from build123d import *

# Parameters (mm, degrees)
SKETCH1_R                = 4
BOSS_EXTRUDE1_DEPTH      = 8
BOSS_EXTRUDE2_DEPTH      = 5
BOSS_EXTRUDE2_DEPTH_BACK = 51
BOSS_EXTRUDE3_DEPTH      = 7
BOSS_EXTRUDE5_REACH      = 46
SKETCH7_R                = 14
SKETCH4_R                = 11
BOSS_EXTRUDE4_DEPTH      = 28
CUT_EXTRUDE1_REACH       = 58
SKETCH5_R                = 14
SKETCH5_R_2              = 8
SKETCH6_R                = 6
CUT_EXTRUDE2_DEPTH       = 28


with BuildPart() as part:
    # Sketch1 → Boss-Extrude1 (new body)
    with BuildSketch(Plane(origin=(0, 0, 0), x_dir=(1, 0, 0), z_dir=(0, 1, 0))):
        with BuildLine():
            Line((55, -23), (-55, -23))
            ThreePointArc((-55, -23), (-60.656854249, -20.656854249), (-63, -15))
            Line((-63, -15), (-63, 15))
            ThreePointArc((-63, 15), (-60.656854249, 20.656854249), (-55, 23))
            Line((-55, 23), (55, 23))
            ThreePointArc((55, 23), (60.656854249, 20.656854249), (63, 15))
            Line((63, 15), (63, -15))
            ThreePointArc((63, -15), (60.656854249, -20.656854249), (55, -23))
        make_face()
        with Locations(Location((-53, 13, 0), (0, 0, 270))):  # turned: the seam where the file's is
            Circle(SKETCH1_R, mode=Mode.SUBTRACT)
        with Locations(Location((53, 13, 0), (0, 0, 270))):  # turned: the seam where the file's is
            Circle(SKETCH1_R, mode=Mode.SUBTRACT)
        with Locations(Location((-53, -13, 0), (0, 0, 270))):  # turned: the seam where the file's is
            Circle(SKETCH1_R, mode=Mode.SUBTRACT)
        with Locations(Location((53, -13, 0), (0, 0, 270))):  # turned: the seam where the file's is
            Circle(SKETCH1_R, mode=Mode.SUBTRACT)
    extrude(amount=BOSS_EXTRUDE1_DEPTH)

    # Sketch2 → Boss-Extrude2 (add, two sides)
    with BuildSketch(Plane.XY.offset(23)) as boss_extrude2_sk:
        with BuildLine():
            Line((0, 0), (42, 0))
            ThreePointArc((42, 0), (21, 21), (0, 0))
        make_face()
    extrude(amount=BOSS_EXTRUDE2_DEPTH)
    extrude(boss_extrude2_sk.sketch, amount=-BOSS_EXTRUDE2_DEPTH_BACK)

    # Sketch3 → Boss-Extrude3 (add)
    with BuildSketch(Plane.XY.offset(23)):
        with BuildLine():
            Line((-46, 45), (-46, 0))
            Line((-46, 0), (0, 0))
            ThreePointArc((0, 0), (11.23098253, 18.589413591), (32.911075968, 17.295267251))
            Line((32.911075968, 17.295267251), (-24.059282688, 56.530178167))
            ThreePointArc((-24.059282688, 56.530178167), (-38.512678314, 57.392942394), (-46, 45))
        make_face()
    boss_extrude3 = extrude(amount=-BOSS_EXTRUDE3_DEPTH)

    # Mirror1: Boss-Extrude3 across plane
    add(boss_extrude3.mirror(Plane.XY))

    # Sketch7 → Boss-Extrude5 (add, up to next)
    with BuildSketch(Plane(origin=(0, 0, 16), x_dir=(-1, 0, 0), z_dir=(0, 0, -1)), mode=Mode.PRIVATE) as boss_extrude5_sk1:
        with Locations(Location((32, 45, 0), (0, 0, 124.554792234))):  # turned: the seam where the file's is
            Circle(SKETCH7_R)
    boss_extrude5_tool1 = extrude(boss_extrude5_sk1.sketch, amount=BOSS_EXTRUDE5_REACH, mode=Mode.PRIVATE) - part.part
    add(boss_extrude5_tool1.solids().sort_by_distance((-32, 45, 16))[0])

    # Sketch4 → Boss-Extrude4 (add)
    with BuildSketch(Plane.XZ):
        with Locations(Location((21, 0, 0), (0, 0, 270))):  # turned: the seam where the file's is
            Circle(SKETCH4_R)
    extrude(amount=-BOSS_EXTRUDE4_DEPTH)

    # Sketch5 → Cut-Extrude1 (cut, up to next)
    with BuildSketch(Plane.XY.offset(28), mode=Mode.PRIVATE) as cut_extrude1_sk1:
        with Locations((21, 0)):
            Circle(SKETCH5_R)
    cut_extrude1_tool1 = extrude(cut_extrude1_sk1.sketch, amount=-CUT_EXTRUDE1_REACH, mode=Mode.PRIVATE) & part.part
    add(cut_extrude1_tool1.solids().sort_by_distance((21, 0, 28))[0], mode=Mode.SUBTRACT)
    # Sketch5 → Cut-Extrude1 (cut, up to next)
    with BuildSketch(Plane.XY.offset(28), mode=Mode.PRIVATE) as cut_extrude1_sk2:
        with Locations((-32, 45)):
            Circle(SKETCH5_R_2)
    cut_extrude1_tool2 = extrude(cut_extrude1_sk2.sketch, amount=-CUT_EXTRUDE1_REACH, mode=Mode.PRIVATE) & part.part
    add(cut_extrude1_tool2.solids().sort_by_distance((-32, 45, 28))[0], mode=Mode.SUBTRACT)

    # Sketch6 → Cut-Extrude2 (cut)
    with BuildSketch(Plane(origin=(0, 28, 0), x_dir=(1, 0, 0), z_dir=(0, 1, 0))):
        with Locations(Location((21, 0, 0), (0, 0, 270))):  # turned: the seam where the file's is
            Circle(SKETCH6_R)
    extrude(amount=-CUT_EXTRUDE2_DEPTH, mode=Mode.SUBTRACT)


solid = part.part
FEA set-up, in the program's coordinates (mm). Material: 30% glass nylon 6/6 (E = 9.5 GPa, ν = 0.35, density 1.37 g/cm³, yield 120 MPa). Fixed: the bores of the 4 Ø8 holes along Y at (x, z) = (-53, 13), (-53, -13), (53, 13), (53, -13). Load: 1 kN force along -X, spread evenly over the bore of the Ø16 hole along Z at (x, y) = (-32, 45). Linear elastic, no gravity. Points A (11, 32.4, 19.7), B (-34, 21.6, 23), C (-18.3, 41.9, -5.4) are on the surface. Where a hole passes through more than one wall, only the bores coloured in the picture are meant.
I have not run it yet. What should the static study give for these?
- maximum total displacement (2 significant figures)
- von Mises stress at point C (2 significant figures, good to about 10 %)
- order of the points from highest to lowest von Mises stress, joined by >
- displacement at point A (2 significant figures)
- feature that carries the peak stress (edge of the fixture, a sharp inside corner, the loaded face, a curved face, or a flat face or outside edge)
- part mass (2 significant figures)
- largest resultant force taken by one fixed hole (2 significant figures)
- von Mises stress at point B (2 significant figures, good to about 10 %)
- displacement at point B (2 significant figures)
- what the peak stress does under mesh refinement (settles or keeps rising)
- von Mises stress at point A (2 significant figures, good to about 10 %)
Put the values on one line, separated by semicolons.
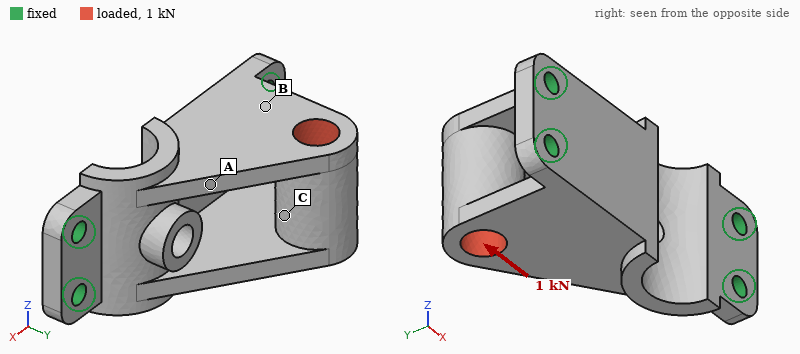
65 µm; 3.2 MPa; A > C > B; 27 µm; edge of the fixture; 130 g; 400 N; 1.1 MPa; 14 µm; keeps rising; 5.4 MPa
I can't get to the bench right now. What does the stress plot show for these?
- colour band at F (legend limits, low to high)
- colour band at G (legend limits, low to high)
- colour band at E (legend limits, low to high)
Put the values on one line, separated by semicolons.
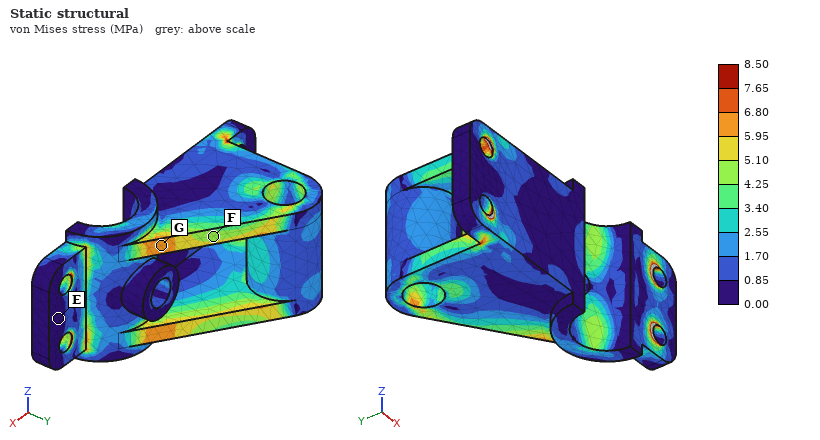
4.25 to 5.10 MPa; 5.95 to 6.80 MPa; 0.00 to 0.85 MPa
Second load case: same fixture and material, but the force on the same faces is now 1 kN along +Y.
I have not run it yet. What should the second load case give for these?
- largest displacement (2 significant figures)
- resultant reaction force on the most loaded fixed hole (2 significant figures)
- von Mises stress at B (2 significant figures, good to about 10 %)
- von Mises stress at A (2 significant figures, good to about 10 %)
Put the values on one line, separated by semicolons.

44 µm; 440 N; 1.9 MPa; 1.4 MPa
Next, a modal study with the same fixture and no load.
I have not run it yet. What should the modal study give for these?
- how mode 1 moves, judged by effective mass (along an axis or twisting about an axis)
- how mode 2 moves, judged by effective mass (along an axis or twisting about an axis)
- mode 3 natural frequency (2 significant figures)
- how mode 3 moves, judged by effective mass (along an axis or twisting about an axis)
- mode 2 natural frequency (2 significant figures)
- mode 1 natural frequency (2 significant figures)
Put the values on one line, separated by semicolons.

along Z; along Y; 3700 Hz; along X; 2900 Hz; 1400 Hz
